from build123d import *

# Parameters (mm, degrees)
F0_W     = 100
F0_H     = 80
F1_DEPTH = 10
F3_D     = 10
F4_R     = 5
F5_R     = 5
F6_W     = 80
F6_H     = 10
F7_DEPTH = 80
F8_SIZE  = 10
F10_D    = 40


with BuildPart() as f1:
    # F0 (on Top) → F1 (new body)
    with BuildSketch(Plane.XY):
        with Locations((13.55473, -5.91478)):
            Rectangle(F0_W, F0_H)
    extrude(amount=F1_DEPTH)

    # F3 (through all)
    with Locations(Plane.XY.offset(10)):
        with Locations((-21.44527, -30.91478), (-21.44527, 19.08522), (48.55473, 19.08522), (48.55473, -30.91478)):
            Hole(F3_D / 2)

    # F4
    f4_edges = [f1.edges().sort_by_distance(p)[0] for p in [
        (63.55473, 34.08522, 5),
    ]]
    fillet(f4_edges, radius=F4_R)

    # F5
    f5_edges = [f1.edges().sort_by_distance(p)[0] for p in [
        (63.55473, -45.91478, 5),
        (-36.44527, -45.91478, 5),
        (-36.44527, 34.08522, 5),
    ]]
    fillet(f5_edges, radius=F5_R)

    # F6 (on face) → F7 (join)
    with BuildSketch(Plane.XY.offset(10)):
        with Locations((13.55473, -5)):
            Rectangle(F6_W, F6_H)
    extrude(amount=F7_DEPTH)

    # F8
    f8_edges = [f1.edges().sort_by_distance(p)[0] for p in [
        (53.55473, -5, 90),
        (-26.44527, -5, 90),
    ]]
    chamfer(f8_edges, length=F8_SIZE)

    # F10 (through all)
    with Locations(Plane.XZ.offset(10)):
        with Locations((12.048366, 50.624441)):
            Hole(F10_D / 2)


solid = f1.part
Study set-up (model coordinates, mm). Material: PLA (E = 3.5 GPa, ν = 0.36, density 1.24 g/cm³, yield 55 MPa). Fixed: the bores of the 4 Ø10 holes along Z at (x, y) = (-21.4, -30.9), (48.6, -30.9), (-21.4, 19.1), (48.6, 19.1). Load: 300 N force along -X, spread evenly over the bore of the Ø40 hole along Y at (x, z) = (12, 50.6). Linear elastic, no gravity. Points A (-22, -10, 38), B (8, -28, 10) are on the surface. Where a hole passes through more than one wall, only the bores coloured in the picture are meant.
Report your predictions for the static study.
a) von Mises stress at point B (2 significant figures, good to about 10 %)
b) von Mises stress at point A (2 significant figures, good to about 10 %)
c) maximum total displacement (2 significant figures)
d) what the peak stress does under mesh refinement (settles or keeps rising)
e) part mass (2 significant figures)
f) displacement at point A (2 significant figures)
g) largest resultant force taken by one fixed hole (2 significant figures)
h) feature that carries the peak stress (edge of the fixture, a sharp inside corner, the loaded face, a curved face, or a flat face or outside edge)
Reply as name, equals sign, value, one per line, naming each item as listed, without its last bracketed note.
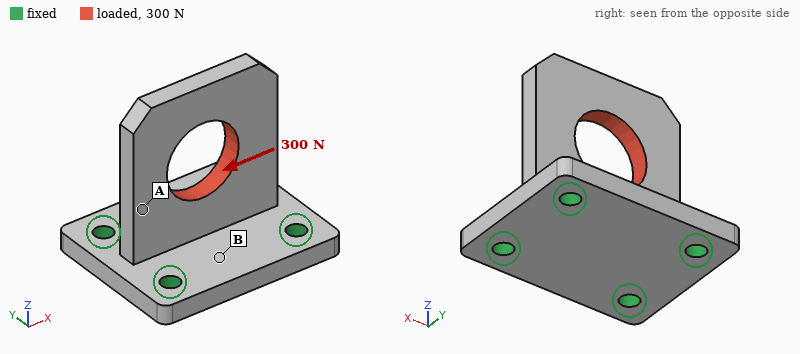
von Mises stress at point B = 0.37 MPa
von Mises stress at point A = 0.89 MPa
maximum total displacement = 92 µm
what the peak stress does under mesh refinement = keeps rising
part mass = 160 g
displacement at point A = 39 µm
largest resultant force taken by one fixed hole = 130 N
feature that carries the peak stress = edge of the fixture
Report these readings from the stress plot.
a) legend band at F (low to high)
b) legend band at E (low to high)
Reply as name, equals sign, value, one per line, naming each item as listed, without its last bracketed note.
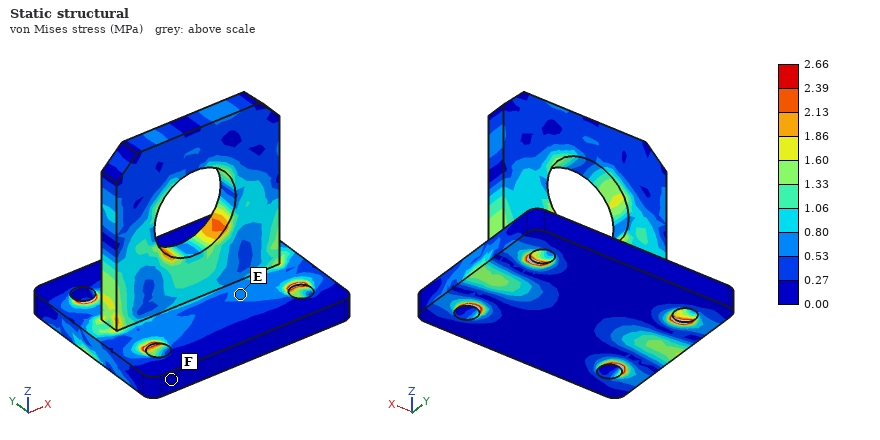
legend band at F = 0.00 to 0.27 MPa
legend band at E = 0.53 to 0.80 MPa
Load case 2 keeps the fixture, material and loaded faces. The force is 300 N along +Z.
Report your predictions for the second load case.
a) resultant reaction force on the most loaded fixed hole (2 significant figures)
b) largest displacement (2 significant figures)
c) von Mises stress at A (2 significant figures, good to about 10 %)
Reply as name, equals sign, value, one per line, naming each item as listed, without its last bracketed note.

resultant reaction force on the most loaded fixed hole = 83 N
largest displacement = 23 µm
von Mises stress at A = 0.50 MPa
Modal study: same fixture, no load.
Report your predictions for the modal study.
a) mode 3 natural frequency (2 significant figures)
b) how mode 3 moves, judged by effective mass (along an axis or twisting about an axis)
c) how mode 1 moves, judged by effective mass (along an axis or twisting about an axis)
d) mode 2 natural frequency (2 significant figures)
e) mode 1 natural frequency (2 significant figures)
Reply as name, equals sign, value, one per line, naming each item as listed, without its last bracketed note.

mode 3 natural frequency = 1300 Hz
how mode 3 moves, judged by effective mass = along X
how mode 1 moves, judged by effective mass = along Y
mode 2 natural frequency = 860 Hz
mode 1 natural frequency = 370 Hz
